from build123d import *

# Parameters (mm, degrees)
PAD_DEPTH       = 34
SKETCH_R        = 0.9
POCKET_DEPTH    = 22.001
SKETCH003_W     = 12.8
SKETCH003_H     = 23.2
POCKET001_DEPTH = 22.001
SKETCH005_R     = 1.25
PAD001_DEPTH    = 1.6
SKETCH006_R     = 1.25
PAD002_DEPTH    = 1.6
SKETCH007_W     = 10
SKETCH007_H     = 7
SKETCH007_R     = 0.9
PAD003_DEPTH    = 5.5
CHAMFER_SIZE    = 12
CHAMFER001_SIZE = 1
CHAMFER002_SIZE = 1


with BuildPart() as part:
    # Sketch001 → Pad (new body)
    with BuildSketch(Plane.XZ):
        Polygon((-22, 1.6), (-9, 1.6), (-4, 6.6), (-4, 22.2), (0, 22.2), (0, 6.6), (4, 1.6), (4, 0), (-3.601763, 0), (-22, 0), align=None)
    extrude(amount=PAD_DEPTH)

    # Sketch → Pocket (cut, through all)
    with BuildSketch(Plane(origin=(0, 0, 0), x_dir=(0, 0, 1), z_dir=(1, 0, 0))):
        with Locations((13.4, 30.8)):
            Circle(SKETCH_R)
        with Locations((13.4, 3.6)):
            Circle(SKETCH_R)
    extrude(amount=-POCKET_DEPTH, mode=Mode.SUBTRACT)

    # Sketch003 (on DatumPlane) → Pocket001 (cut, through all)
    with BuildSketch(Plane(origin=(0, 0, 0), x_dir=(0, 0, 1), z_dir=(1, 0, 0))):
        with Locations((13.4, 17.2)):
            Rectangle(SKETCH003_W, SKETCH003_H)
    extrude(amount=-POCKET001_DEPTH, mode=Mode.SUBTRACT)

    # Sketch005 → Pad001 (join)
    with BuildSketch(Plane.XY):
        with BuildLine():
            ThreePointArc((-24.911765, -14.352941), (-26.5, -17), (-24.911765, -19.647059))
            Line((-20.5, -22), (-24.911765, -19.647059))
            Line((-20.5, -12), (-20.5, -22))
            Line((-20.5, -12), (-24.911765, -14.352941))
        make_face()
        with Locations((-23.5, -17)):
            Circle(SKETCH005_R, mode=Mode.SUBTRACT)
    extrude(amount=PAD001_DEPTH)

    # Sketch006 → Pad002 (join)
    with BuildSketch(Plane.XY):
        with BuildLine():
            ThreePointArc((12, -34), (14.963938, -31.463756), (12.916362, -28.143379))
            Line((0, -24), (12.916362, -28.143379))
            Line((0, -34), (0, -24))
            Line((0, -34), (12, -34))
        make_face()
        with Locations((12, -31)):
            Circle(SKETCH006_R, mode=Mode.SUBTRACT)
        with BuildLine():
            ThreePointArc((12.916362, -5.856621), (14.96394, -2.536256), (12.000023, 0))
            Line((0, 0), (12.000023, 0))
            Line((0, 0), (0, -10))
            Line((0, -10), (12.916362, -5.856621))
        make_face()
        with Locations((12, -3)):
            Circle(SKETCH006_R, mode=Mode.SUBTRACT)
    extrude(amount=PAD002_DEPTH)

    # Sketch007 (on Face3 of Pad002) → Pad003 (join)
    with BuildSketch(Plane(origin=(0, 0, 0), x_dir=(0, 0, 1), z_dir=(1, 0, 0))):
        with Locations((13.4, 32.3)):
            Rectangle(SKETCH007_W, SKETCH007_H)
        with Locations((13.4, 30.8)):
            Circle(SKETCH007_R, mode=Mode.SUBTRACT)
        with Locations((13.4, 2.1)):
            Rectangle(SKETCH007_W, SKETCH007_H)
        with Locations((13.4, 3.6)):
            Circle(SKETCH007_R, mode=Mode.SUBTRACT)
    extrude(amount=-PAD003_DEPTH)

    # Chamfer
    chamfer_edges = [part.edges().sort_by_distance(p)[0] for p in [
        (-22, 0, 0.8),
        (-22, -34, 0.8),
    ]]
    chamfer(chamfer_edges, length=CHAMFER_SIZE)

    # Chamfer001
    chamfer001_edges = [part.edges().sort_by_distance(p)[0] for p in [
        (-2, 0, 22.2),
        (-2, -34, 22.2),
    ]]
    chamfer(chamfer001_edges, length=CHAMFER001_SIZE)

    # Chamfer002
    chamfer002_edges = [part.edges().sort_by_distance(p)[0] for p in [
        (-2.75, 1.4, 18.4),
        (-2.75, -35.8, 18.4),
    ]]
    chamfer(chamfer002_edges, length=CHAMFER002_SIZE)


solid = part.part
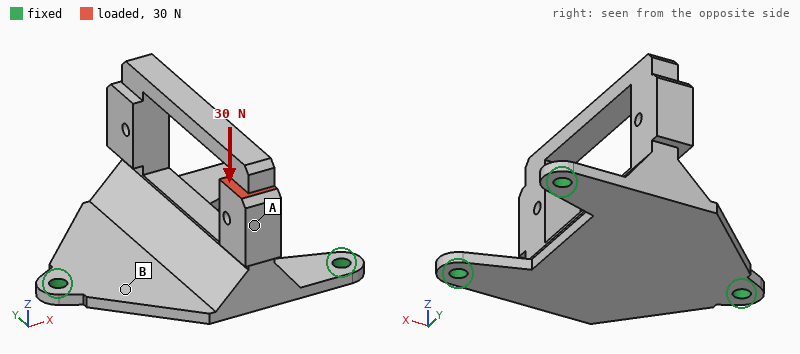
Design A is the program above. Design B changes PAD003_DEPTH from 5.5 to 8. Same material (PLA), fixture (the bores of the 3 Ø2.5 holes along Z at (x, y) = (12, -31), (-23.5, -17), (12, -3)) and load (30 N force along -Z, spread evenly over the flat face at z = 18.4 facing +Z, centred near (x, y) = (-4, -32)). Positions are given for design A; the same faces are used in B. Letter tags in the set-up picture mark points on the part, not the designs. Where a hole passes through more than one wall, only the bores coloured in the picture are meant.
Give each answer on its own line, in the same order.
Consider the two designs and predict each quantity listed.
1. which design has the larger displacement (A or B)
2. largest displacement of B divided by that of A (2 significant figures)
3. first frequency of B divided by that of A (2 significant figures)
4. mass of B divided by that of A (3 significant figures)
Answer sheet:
B
1.1
0.92
1.08
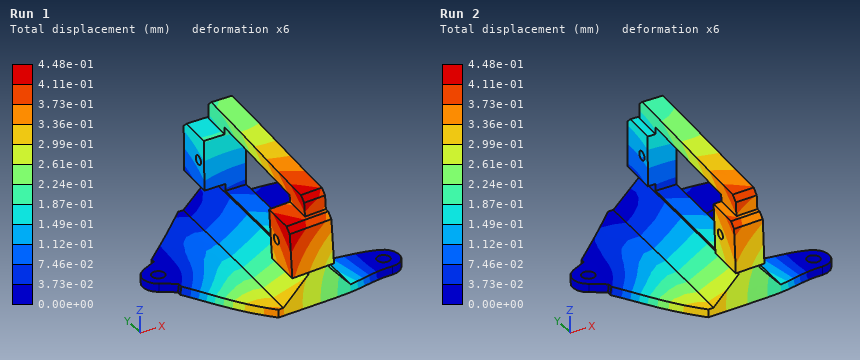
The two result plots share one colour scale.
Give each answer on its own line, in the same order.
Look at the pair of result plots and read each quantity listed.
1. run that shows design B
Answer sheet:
Run 1
